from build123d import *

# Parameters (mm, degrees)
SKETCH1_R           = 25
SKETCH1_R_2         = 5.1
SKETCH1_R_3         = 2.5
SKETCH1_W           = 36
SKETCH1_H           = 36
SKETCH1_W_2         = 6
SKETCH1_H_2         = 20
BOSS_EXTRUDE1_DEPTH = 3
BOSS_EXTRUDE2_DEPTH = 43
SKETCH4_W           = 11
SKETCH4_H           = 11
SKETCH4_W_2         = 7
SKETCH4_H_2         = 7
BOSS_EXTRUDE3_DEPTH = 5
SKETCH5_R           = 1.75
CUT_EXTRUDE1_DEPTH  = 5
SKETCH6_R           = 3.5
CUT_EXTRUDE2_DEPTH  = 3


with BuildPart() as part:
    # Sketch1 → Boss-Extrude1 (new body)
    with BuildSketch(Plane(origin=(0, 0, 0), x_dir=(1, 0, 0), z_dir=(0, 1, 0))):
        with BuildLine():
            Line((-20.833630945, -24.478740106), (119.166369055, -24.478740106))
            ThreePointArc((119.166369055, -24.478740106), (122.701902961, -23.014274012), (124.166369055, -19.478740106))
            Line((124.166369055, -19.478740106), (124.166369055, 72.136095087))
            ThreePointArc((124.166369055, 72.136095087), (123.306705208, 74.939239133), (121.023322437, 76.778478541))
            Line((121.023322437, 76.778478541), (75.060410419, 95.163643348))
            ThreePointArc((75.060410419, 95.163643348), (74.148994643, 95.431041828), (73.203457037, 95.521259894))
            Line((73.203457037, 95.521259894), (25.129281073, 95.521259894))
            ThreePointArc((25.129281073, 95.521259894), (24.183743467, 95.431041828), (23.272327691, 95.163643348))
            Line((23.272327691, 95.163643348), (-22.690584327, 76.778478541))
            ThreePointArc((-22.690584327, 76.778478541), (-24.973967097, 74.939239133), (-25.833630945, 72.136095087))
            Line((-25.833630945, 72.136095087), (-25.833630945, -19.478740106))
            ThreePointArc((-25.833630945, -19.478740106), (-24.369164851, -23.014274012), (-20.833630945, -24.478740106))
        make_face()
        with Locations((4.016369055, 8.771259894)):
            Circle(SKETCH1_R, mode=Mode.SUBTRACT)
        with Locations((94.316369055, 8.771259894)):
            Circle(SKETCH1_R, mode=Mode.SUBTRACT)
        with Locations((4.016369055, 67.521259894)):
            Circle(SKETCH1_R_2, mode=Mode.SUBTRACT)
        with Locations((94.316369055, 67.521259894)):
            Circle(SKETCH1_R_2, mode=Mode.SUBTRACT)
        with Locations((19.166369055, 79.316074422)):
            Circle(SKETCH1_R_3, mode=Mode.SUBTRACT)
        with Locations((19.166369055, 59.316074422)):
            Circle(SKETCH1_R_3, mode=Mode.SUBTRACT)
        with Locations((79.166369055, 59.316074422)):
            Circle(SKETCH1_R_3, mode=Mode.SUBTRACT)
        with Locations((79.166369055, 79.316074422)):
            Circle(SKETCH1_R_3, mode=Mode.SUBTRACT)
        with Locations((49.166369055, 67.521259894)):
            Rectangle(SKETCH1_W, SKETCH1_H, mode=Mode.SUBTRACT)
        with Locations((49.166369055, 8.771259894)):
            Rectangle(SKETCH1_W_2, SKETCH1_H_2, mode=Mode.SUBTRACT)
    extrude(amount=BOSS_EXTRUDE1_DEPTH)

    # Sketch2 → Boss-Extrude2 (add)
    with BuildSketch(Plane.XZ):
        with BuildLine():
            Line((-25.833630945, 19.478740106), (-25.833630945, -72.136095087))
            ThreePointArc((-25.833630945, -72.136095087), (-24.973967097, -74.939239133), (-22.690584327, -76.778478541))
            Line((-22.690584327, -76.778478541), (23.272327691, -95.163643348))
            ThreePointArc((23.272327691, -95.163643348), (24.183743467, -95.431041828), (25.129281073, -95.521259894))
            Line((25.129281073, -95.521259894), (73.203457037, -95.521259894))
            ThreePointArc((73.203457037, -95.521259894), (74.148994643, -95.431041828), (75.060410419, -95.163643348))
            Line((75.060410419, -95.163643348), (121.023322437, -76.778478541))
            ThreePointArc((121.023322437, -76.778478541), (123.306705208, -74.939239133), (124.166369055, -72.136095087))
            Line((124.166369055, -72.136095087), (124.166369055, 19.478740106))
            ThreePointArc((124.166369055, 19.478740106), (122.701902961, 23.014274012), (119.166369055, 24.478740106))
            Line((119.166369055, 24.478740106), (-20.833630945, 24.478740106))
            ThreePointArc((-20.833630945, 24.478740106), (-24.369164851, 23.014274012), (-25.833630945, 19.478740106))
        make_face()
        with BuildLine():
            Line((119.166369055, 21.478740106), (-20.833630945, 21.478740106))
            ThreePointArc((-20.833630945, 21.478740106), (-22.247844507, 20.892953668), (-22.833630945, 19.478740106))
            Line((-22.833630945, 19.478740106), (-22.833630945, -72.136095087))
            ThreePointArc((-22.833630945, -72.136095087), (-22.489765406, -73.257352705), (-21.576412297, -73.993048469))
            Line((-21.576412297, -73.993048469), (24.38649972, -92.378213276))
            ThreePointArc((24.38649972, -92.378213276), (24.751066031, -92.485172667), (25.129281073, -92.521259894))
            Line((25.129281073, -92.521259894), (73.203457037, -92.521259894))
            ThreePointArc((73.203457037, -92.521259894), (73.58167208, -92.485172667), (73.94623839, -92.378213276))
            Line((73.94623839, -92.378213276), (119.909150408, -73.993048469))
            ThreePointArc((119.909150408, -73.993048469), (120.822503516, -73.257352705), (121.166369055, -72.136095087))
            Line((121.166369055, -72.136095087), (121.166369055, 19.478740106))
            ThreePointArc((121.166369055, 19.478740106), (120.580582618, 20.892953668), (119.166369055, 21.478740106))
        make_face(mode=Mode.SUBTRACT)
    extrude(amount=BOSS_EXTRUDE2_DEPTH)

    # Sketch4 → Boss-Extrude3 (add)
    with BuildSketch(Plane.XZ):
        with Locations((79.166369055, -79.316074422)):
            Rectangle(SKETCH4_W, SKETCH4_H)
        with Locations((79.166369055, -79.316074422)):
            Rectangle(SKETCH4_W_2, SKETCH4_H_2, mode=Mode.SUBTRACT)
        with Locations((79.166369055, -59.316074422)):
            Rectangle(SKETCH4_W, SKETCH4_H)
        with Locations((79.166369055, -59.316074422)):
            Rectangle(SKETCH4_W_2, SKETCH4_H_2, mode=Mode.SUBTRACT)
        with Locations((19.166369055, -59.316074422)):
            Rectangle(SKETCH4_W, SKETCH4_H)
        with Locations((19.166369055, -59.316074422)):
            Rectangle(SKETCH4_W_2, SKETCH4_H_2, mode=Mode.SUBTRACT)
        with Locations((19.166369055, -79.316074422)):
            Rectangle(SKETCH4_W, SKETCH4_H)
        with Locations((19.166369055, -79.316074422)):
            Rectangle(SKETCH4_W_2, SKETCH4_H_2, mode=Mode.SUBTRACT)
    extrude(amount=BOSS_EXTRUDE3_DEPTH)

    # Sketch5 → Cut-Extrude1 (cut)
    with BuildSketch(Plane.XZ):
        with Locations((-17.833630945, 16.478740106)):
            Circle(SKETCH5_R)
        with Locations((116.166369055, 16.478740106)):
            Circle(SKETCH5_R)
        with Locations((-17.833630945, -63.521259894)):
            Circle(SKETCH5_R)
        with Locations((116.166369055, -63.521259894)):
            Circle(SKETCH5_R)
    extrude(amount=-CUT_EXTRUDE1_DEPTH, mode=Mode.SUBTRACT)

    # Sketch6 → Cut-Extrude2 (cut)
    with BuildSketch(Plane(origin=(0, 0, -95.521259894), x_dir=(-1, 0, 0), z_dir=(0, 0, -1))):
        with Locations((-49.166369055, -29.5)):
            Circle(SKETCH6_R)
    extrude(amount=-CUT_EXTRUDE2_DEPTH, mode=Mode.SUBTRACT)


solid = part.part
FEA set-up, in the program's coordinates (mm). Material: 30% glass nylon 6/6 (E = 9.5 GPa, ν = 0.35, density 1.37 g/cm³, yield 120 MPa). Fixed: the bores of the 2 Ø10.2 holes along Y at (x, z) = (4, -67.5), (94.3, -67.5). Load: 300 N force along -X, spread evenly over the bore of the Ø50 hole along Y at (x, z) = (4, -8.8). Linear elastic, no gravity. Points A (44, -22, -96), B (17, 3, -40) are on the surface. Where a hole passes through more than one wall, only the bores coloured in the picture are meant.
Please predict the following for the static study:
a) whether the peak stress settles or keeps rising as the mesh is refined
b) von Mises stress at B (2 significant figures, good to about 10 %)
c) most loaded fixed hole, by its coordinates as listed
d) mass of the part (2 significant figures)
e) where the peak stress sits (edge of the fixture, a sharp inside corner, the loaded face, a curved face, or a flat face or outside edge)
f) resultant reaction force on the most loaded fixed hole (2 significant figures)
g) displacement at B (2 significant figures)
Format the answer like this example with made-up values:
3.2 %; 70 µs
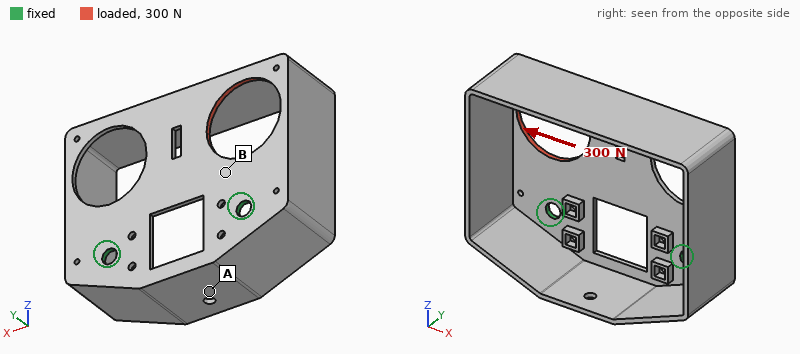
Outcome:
keeps rising; 3.1 MPa; (4, -67.5); 140 g; edge of the fixture; 240 N; 18 µm
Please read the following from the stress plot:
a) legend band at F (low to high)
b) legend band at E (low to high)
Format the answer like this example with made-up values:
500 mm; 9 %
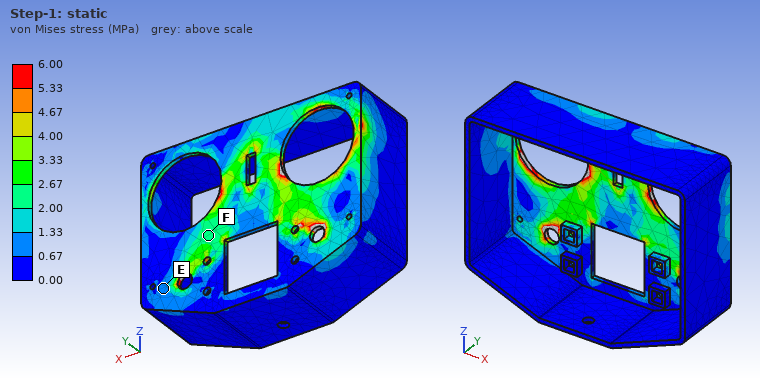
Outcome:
2.00 to 2.67 MPa; 0.67 to 1.33 MPa
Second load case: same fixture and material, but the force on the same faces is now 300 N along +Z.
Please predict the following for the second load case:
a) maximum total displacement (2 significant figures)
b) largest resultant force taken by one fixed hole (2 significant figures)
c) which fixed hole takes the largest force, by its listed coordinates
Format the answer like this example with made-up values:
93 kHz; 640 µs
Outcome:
56 µm; 290 N; (4, -67.5)
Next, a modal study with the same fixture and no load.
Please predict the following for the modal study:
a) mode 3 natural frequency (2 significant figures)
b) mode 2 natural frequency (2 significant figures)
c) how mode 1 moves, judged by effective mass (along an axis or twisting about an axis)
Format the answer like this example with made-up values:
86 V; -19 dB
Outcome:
520 Hz; 220 Hz; along Y
